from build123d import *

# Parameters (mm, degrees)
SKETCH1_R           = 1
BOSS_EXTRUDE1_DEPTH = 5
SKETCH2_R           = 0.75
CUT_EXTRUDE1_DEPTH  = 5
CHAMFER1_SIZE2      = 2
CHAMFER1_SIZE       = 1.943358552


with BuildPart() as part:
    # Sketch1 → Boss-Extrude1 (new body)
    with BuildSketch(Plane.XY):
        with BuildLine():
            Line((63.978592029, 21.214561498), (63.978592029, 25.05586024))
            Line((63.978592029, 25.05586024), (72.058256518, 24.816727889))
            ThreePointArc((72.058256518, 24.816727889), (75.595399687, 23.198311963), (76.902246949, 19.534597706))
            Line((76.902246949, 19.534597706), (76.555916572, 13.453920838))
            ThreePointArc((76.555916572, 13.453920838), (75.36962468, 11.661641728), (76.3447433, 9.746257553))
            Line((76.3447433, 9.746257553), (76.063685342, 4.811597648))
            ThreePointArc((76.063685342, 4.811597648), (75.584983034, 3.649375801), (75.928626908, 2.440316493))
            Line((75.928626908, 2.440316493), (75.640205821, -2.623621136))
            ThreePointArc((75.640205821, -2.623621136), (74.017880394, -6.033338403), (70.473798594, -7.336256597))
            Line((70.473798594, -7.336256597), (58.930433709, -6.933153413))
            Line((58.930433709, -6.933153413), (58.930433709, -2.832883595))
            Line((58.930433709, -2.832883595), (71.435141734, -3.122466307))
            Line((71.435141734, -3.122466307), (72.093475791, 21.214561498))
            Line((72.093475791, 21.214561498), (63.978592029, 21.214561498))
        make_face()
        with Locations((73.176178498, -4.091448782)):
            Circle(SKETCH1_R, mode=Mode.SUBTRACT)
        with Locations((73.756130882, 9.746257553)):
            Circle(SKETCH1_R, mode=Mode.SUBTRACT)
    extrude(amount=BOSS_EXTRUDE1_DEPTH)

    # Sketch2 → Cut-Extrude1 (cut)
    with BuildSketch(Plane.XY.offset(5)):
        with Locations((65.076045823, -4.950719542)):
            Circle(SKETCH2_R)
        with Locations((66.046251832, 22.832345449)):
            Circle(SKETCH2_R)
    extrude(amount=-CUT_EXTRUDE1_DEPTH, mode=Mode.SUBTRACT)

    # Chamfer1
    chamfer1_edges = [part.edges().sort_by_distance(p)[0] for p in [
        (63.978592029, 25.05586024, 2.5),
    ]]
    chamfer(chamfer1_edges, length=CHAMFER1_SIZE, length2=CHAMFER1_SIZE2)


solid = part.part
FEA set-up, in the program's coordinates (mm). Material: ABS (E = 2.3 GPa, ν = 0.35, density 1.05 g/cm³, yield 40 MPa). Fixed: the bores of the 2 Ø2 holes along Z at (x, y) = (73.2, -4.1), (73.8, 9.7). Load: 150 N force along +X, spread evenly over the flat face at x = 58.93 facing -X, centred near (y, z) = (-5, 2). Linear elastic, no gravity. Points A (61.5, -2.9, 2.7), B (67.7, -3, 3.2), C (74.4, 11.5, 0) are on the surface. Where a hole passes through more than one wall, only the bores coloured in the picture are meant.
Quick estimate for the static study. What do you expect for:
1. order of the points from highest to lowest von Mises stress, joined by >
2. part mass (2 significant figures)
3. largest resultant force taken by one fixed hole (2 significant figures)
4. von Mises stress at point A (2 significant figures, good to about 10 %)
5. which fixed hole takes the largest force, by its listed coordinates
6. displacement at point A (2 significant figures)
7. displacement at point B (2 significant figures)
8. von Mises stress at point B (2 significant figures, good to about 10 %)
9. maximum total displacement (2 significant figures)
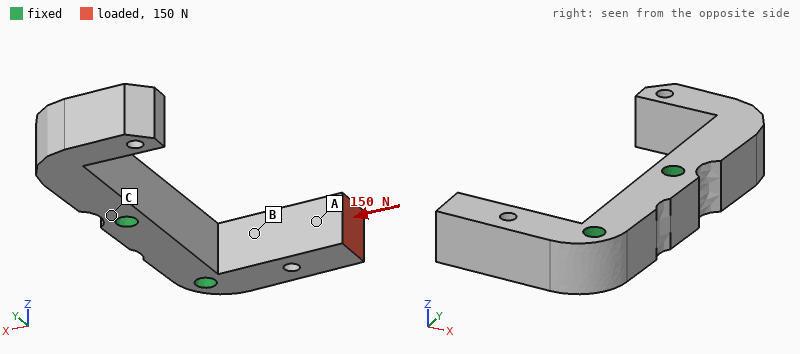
B > A > C
1.1 g
150 N
8.5 MPa
(73.2, -4.1)
47 µm
20 µm
11 MPa
55 µm
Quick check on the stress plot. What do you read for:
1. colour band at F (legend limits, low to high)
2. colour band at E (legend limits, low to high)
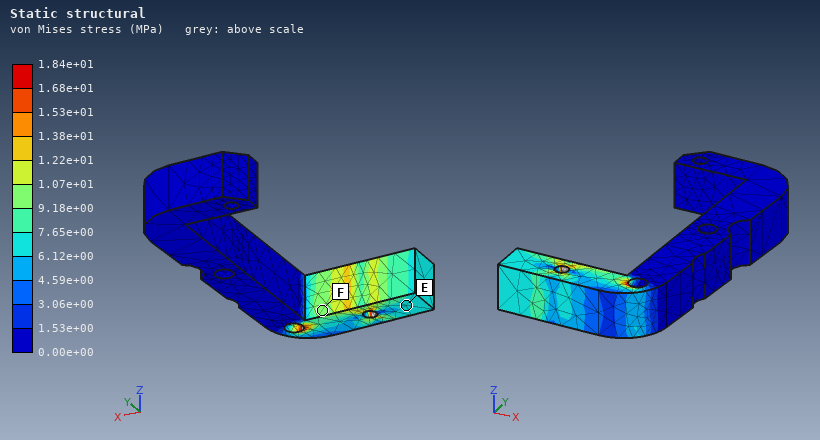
9.18e+00 to 1.07e+01 MPa
6.12e+00 to 7.65e+00 MPa
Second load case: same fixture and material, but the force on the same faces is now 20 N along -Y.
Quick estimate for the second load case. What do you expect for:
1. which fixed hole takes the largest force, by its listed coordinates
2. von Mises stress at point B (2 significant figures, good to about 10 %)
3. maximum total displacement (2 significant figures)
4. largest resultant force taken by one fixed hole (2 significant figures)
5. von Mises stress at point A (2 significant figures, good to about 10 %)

(73.2, -4.1)
12 MPa
0.34 mm
18 N
3.6 MPa
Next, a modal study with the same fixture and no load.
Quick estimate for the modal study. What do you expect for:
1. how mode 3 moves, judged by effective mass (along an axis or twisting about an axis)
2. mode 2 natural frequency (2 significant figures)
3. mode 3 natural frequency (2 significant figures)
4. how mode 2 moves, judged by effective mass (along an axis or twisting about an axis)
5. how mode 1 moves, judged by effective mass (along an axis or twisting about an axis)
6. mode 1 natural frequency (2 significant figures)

along Y
3000 Hz
4400 Hz
along Z
along X
2400 Hz
